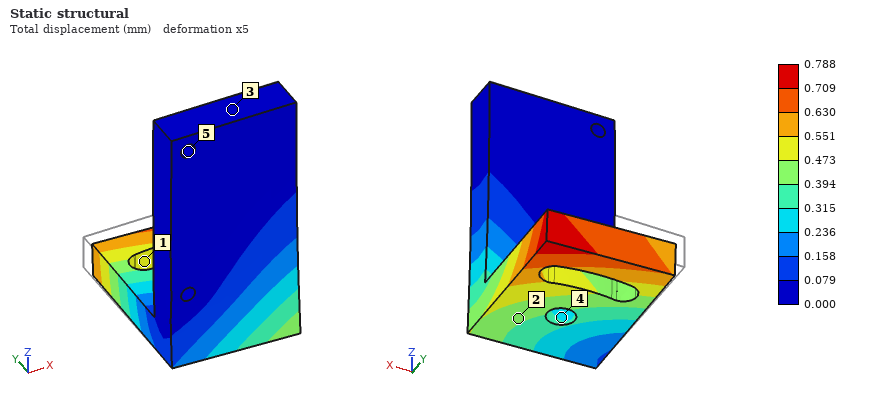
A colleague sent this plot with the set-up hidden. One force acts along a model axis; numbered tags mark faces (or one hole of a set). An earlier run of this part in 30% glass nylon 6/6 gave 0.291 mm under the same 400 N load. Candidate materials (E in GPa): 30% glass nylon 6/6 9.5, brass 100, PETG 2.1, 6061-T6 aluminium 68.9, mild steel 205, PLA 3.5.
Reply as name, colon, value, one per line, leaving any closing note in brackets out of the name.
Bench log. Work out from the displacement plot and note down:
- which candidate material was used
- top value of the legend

which candidate material was used: PLA
top value of the legend: 0.788 mm
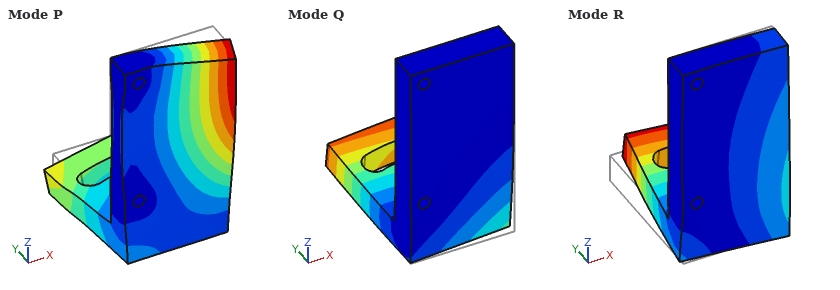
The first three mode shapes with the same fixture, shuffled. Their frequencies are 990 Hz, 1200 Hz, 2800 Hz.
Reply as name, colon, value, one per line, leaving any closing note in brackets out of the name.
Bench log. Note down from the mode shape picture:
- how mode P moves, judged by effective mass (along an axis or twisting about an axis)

how mode P moves, judged by effective mass: along Y
